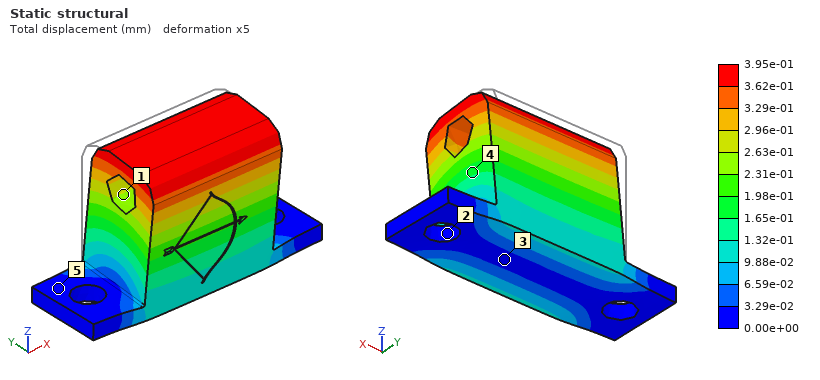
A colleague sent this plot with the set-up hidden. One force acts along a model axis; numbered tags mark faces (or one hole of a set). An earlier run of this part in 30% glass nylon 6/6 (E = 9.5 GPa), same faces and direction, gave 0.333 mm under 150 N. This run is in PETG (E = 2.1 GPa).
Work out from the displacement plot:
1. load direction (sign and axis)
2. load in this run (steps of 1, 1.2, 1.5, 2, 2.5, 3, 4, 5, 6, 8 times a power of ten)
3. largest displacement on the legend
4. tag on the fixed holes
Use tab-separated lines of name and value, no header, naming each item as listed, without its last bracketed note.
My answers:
load direction	-Y
load in this run	40 N
largest displacement on the legend	3.95e-01 mm
tag on the fixed holes	2
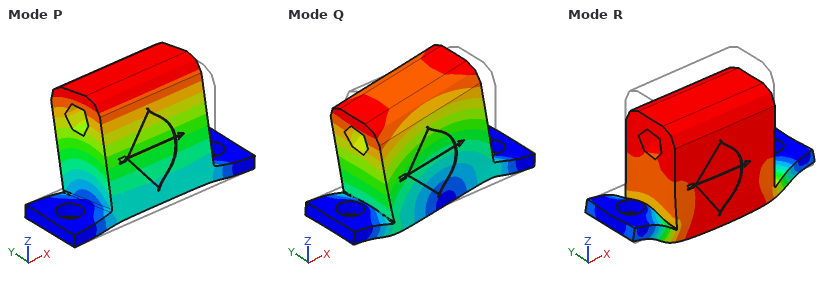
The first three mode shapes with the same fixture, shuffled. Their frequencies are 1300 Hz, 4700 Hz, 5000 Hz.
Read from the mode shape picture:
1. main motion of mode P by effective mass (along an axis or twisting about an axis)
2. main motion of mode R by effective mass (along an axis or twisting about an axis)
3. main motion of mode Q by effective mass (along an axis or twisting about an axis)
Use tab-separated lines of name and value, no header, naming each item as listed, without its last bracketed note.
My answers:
main motion of mode P by effective mass	along Y
main motion of mode R by effective mass	along Z
main motion of mode Q by effective mass	along X
